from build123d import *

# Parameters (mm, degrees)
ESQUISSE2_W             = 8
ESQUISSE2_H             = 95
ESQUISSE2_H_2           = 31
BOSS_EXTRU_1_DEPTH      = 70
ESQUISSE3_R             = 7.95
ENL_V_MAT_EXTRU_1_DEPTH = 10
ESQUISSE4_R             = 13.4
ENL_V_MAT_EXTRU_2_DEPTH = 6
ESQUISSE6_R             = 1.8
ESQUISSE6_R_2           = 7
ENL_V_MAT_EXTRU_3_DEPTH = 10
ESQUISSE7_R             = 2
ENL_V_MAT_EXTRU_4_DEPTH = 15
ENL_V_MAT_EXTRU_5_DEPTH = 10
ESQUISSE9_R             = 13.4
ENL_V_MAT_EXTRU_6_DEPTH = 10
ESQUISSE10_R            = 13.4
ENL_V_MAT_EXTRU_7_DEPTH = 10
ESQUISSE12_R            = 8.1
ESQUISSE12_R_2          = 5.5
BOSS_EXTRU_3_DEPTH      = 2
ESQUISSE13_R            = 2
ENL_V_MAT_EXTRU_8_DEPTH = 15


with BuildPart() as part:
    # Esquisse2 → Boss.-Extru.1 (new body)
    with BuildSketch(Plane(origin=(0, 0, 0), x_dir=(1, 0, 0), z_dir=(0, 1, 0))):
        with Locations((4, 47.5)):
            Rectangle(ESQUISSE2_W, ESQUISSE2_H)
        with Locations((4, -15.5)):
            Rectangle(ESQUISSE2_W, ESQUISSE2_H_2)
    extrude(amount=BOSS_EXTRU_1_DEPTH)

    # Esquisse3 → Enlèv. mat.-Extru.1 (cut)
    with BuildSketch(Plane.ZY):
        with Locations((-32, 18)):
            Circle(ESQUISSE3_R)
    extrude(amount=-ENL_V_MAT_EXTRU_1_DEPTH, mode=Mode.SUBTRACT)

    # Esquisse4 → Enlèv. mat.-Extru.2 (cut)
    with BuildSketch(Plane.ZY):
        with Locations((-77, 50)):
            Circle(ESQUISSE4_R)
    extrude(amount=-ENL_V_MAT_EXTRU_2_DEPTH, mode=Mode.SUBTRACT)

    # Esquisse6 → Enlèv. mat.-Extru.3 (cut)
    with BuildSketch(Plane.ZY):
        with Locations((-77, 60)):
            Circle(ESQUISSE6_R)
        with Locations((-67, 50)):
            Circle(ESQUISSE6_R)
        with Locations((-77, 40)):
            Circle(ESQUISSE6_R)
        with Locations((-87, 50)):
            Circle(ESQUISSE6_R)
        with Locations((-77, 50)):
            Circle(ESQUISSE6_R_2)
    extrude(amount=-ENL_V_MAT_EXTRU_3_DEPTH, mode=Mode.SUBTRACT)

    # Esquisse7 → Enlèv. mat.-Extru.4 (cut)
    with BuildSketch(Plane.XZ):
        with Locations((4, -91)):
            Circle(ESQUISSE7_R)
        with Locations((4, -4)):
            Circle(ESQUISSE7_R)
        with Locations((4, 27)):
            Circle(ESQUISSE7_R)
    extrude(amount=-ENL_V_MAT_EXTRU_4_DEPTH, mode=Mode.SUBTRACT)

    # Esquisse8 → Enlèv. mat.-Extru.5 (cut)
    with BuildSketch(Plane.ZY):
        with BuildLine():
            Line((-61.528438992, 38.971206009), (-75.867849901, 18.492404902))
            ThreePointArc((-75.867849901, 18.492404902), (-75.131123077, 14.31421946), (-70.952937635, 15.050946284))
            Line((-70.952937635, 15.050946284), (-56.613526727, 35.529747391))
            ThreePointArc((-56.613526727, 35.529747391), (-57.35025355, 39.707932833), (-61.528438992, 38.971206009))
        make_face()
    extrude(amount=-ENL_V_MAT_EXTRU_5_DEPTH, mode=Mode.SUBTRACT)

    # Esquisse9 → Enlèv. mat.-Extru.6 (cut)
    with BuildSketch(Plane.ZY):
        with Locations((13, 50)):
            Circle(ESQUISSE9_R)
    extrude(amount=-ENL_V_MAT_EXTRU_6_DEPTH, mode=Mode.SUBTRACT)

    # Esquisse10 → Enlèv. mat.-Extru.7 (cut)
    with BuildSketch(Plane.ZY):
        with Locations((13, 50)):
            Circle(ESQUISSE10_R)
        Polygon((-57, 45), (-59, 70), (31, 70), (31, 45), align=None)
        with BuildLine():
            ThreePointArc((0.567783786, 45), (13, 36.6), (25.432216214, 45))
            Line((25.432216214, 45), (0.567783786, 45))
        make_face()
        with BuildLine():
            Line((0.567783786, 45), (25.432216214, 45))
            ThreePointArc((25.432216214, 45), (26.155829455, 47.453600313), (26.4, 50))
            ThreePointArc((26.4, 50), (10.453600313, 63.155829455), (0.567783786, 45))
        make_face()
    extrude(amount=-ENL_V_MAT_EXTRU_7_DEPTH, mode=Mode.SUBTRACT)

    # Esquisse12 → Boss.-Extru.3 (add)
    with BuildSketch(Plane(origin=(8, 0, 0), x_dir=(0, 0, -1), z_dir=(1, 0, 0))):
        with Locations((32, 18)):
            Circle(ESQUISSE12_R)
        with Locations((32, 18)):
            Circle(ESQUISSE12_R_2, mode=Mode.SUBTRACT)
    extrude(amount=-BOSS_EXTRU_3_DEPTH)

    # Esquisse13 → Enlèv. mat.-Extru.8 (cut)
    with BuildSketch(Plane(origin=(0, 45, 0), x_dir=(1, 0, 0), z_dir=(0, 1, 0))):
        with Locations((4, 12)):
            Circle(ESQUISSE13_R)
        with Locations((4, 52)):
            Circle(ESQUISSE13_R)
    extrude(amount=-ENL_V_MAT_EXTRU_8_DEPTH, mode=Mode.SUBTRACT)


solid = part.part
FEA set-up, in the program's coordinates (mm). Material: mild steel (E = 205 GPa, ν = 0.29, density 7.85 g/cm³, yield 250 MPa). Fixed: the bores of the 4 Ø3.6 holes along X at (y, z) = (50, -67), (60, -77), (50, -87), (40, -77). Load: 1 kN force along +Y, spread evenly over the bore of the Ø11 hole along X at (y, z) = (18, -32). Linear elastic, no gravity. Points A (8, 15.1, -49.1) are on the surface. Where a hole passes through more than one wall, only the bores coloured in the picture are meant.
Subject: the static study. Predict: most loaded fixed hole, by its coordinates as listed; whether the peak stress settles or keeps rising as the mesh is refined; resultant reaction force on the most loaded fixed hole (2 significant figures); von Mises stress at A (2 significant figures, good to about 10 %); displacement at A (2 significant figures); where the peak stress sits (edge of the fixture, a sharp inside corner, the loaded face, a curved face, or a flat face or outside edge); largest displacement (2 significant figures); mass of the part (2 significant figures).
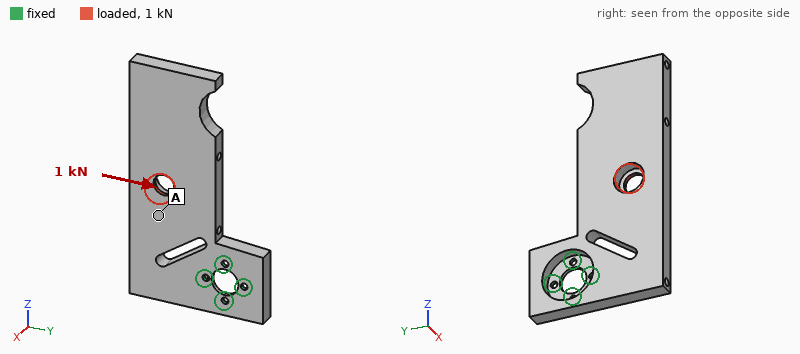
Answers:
(50, -67)
keeps rising
1.6 kN
10 MPa
15 µm
edge of the fixture
43 µm
350 g
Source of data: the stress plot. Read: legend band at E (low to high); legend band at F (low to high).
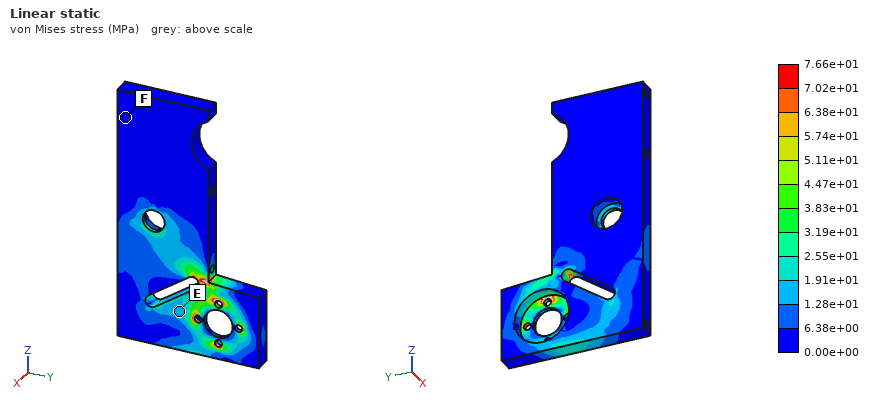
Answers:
1.28e+01 to 1.91e+01 MPa
0.00e+00 to 6.38e+00 MPa
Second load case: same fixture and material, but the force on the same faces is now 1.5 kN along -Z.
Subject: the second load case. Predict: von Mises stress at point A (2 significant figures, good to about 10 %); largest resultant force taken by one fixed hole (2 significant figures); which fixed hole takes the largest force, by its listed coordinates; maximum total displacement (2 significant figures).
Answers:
15 MPa
1.6 kN
(40, -77)
98 µm
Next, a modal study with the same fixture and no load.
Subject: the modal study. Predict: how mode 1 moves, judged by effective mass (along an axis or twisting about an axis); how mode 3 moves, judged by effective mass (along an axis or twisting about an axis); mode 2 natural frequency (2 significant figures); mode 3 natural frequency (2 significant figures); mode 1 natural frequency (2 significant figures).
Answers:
along X
along Y
1400 Hz
1500 Hz
360 Hz
